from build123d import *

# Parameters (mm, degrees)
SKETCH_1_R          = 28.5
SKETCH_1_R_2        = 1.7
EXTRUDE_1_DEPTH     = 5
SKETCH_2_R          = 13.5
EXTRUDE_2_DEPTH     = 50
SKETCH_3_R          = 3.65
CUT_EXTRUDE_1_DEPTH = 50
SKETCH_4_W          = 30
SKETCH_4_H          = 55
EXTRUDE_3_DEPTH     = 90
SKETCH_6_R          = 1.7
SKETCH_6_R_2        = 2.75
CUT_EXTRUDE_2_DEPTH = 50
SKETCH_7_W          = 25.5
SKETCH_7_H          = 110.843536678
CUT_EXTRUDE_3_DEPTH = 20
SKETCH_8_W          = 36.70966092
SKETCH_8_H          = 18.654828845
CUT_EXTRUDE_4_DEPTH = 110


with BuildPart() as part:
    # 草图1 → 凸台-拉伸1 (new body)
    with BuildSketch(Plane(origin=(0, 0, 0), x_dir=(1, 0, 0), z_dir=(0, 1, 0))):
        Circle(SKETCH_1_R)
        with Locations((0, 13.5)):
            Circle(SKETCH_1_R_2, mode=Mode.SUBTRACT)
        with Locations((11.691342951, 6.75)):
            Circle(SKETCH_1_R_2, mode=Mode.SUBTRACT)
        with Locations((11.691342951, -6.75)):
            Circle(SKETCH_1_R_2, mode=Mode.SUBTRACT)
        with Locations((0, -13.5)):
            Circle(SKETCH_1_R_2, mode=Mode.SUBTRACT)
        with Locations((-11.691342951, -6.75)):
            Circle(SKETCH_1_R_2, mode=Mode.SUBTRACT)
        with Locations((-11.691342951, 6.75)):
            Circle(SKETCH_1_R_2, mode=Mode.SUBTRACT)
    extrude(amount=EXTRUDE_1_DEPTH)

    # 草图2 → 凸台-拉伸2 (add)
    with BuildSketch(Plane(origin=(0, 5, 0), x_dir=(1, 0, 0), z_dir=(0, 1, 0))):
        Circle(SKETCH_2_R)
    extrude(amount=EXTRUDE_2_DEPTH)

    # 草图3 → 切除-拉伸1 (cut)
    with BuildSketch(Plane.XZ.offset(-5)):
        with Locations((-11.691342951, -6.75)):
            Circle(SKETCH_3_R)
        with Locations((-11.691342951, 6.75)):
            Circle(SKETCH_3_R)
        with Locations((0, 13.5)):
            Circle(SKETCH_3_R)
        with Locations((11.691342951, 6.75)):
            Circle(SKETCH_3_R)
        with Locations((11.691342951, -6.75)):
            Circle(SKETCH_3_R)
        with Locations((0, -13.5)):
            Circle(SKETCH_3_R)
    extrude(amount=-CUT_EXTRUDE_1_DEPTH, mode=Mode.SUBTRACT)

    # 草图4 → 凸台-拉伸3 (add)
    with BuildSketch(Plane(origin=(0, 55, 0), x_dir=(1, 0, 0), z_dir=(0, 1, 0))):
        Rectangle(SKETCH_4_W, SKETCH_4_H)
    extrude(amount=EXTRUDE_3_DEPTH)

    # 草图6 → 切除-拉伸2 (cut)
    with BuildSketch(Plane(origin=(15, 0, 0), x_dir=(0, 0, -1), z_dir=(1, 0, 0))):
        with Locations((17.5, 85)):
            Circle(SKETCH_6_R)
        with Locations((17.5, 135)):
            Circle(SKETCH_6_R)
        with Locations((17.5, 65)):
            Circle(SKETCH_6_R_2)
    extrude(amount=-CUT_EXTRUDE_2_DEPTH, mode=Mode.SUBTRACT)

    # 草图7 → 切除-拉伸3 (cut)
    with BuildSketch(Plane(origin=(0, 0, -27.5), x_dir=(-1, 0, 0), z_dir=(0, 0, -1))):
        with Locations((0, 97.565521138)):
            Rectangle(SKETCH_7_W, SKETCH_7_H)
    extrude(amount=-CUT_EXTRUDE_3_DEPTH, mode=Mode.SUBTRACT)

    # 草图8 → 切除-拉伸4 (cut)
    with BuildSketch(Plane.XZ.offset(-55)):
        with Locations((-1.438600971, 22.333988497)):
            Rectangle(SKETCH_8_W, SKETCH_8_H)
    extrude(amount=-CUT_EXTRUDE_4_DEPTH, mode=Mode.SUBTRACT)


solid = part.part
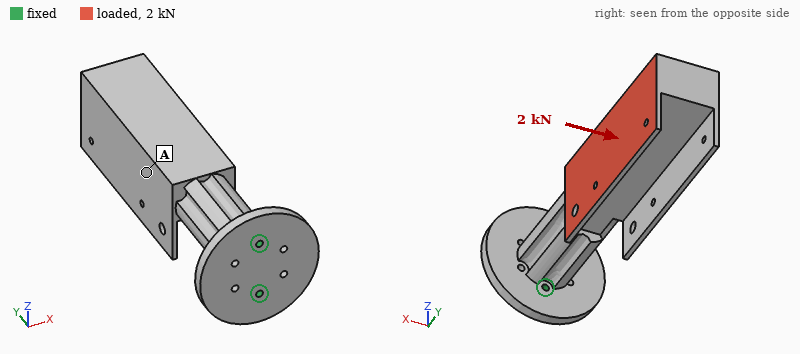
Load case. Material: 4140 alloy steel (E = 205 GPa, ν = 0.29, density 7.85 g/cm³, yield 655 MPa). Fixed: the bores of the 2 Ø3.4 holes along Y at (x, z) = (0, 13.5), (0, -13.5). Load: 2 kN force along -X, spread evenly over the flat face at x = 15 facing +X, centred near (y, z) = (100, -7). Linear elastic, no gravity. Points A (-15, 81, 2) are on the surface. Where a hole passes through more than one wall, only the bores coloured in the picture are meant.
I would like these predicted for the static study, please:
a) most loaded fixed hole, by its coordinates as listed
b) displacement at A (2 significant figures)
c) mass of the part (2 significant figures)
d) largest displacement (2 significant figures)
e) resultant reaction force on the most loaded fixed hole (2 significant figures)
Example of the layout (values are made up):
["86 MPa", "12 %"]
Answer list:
["(0, -13.5)", "0.72 mm", "770 g", "1.4 mm", "1.5 kN"]
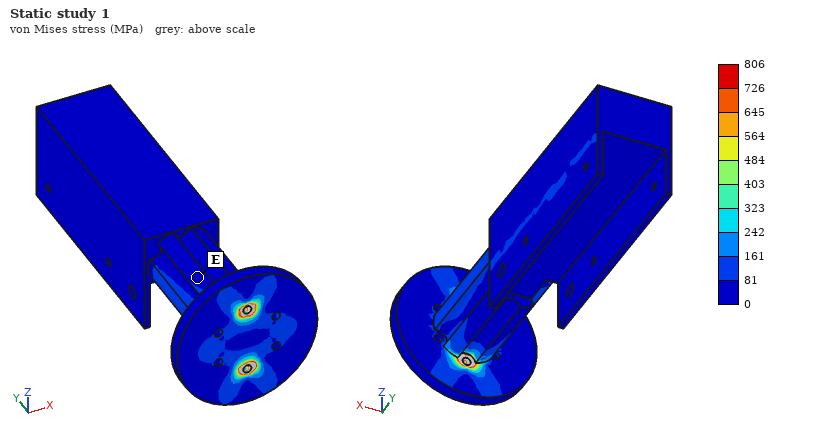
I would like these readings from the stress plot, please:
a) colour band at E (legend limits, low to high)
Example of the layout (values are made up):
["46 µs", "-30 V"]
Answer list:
["0 to 81 MPa"]
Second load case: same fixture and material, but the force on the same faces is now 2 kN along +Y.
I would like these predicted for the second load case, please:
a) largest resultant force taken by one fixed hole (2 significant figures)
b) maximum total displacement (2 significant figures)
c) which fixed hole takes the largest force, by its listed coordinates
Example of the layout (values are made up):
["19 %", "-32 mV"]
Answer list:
["1.6 kN", "0.24 mm", "(0, -13.5)"]
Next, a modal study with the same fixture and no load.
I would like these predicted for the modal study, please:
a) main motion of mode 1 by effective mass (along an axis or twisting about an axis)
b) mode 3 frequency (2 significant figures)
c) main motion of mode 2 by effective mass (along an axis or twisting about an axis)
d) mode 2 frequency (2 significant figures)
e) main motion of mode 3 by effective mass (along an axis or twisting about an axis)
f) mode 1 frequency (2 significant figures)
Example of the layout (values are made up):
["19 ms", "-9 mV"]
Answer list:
["along X", "2600 Hz", "along Z", "590 Hz", "twisting about Y", "320 Hz"]
